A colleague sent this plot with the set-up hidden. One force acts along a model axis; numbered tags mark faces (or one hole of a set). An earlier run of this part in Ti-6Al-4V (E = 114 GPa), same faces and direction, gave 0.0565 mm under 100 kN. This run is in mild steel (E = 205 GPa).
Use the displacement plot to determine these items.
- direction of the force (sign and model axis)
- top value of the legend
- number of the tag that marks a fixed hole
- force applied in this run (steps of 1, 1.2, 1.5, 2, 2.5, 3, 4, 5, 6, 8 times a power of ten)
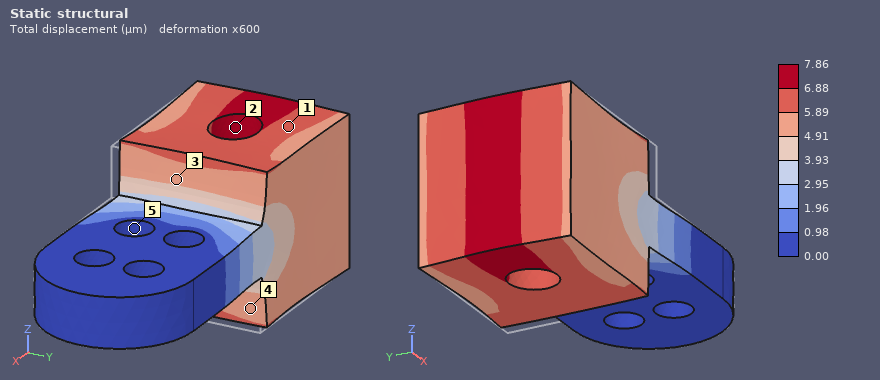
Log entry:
-X
7.86 µm
5
25 kN
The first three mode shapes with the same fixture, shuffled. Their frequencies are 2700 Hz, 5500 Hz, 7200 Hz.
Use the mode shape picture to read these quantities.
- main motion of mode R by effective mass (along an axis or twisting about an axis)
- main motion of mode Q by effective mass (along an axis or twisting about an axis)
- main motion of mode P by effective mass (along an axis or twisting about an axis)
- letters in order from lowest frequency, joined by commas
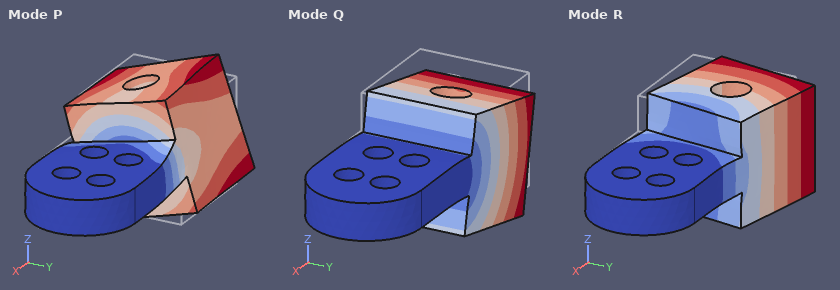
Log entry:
along Y
along Z
twisting about X
Q, R, P
